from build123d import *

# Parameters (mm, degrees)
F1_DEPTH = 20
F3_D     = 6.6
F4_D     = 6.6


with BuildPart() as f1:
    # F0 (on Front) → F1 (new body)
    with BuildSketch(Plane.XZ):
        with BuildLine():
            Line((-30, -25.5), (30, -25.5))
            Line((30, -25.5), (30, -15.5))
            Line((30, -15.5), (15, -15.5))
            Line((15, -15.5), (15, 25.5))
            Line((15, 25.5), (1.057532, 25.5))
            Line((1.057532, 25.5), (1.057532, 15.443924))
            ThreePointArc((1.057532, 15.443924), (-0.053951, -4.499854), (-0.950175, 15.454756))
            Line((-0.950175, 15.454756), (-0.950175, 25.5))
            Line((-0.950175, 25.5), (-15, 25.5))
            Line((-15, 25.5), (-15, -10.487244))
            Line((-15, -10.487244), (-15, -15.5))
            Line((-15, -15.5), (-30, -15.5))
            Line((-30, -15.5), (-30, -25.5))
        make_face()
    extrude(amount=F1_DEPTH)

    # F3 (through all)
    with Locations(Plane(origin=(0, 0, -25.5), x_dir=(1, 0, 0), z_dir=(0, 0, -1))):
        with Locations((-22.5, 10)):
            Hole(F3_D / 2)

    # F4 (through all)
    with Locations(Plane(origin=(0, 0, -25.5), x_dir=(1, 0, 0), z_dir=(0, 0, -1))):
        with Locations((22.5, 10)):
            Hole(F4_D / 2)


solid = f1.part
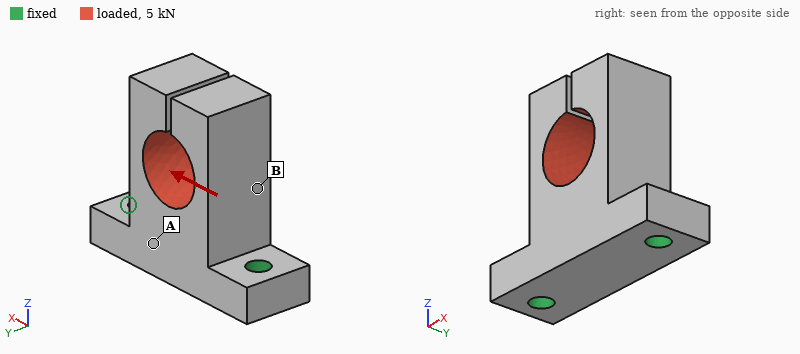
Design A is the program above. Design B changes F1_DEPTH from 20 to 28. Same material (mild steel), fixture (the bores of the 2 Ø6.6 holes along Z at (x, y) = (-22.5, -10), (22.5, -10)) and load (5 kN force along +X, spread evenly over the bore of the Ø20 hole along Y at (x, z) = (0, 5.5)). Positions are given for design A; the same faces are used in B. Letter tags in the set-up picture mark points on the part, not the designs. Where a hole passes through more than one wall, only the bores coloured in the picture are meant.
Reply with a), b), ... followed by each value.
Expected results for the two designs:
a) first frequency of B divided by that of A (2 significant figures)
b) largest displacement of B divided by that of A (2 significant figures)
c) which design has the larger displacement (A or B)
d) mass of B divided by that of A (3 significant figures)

a) 1.00
b) 0.73
c) A
d) 1.41
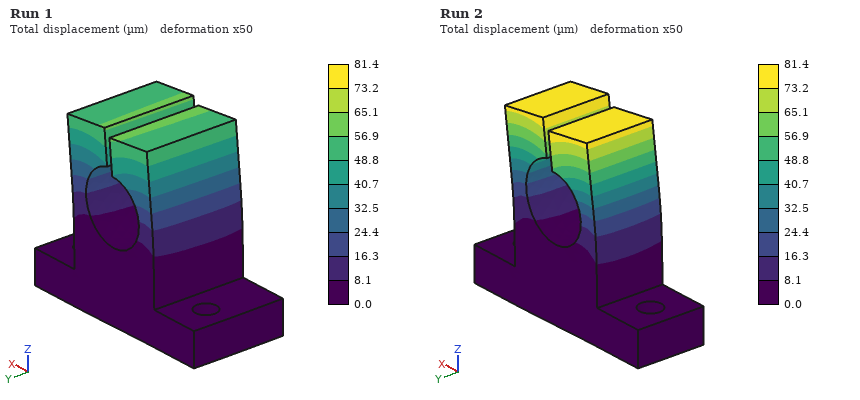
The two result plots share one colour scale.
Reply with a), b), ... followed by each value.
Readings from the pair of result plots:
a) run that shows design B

a) Run 1
